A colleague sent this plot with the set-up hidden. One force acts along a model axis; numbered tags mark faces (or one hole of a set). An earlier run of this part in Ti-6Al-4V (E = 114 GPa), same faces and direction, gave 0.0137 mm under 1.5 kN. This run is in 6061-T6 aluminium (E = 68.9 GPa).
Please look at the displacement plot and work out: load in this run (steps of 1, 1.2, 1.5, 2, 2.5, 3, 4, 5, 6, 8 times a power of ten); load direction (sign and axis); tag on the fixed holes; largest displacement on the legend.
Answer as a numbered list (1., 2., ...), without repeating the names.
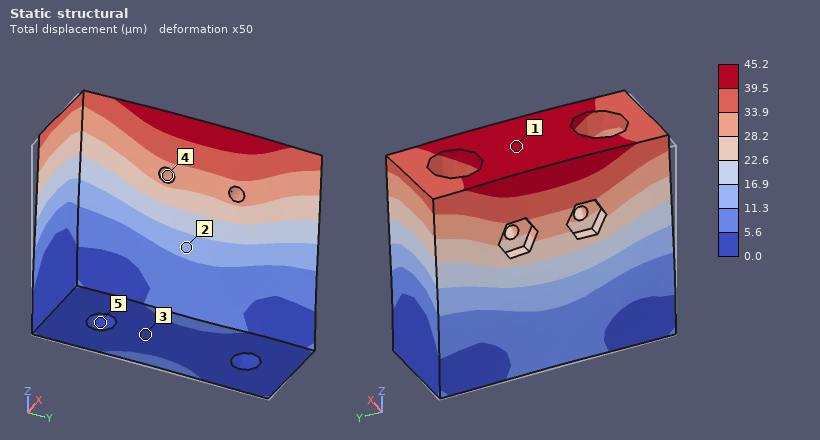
1. 3 kN
2. +X
3. 5
4. 45.2 µm
